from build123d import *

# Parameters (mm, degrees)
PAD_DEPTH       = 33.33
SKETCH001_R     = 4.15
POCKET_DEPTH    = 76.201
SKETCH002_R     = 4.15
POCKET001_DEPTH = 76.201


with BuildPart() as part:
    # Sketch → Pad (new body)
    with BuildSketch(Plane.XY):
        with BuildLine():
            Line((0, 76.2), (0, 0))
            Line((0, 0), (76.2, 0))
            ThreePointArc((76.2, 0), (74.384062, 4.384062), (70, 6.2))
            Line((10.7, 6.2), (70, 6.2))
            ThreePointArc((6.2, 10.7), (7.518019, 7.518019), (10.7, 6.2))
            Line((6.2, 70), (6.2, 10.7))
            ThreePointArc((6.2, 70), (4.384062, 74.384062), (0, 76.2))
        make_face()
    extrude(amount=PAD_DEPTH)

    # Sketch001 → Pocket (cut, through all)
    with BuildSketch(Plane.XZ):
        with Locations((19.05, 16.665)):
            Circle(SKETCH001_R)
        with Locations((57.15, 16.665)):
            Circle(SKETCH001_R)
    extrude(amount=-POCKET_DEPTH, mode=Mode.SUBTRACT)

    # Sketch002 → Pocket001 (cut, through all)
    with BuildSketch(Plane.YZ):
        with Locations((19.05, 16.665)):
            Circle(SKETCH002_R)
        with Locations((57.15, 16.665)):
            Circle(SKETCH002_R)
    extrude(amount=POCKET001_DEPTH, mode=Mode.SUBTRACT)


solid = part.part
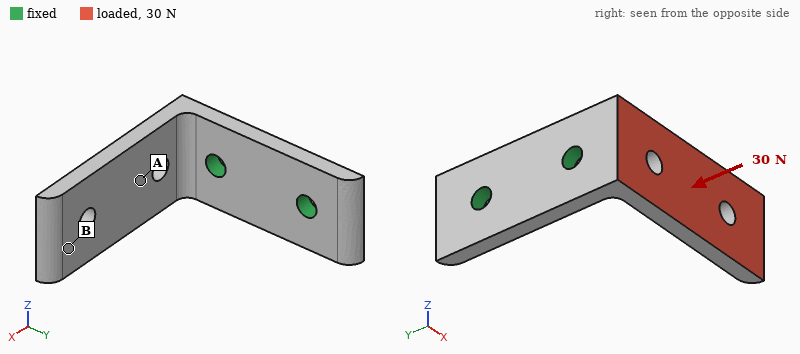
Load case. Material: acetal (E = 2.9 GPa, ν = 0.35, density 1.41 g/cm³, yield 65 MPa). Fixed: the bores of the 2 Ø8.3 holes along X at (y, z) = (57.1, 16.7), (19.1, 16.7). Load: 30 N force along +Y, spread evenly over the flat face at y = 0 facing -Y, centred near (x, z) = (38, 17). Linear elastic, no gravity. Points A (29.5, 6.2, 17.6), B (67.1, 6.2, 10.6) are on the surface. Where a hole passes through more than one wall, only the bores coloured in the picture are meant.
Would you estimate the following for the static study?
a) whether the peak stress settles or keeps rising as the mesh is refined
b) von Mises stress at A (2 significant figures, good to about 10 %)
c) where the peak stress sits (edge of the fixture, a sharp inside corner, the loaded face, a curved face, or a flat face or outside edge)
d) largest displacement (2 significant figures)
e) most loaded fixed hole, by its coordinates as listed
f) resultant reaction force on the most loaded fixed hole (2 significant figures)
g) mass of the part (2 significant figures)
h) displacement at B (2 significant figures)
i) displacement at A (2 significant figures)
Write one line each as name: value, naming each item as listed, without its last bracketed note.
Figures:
whether the peak stress settles or keeps rising as the mesh is refined: keeps rising
von Mises stress at A: 1.6 MPa
where the peak stress sits: edge of the fixture
largest displacement: 1.1 mm
most loaded fixed hole, by its coordinates as listed: (19.1, 16.7)
resultant reaction force on the most loaded fixed hole: 28 N
mass of the part: 40 g
displacement at B: 0.95 mm
displacement at A: 0.28 mm
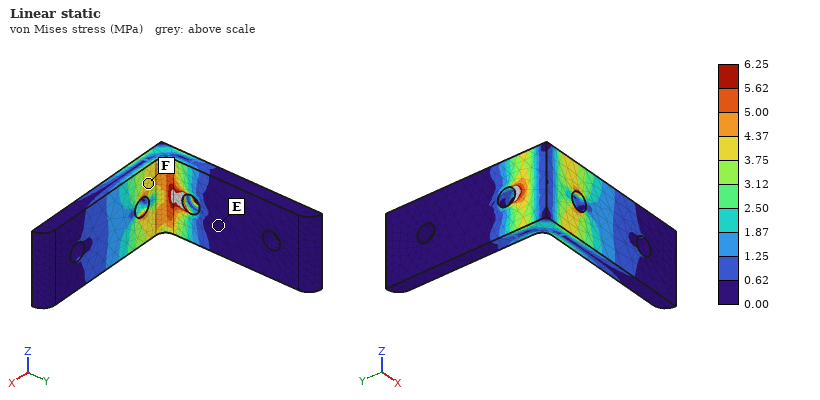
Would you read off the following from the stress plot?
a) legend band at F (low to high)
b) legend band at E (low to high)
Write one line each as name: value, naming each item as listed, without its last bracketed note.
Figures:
legend band at F: 3.75 to 4.37 MPa
legend band at E: 0.00 to 0.62 MPa
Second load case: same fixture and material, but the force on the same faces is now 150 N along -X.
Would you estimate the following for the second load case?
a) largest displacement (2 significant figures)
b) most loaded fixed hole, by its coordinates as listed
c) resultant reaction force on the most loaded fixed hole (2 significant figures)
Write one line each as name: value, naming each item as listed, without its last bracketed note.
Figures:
largest displacement: 1.2 mm
most loaded fixed hole, by its coordinates as listed: (19.1, 16.7)
resultant reaction force on the most loaded fixed hole: 160 N
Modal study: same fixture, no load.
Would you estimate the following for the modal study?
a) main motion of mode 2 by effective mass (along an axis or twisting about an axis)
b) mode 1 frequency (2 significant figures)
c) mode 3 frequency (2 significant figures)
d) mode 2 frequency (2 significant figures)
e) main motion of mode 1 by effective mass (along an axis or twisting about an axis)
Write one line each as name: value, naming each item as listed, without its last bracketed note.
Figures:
main motion of mode 2 by effective mass: along Z
mode 1 frequency: 230 Hz
mode 3 frequency: 1100 Hz
mode 2 frequency: 430 Hz
main motion of mode 1 by effective mass: along Y
